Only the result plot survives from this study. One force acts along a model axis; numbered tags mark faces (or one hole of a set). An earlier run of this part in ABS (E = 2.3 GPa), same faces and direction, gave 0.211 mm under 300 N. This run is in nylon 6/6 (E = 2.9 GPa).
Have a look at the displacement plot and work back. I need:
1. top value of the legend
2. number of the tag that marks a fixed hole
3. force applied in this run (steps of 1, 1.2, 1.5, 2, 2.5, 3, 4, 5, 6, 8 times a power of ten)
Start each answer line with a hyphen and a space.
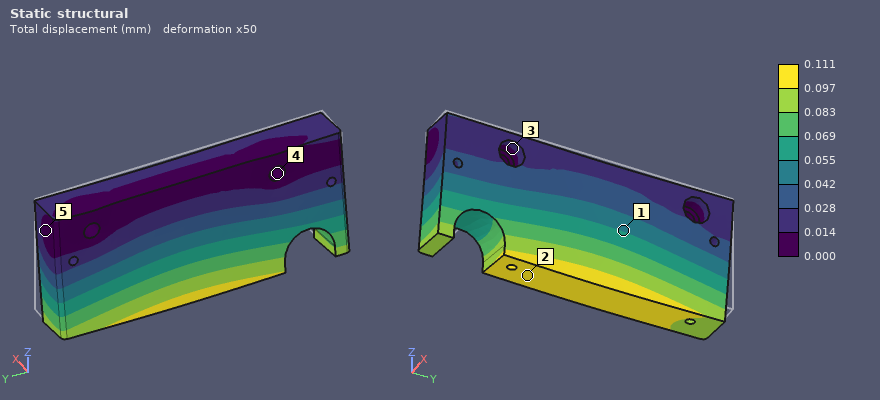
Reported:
- 0.111 mm
- 4
- 200 N
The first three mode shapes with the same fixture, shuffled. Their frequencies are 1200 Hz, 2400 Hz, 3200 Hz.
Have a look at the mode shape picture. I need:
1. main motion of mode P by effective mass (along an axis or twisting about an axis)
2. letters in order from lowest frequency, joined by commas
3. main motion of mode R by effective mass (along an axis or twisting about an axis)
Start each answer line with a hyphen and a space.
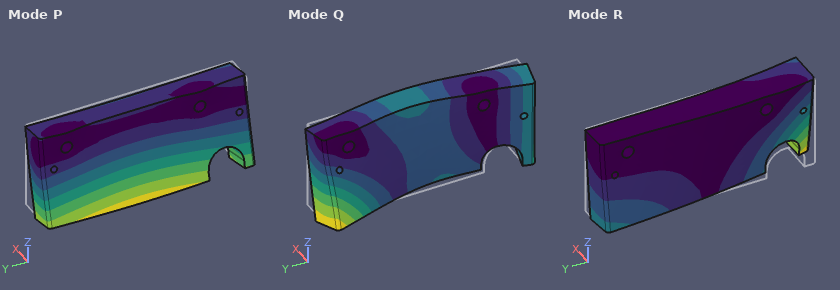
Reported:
- along X
- P, R, Q
- twisting about Z
